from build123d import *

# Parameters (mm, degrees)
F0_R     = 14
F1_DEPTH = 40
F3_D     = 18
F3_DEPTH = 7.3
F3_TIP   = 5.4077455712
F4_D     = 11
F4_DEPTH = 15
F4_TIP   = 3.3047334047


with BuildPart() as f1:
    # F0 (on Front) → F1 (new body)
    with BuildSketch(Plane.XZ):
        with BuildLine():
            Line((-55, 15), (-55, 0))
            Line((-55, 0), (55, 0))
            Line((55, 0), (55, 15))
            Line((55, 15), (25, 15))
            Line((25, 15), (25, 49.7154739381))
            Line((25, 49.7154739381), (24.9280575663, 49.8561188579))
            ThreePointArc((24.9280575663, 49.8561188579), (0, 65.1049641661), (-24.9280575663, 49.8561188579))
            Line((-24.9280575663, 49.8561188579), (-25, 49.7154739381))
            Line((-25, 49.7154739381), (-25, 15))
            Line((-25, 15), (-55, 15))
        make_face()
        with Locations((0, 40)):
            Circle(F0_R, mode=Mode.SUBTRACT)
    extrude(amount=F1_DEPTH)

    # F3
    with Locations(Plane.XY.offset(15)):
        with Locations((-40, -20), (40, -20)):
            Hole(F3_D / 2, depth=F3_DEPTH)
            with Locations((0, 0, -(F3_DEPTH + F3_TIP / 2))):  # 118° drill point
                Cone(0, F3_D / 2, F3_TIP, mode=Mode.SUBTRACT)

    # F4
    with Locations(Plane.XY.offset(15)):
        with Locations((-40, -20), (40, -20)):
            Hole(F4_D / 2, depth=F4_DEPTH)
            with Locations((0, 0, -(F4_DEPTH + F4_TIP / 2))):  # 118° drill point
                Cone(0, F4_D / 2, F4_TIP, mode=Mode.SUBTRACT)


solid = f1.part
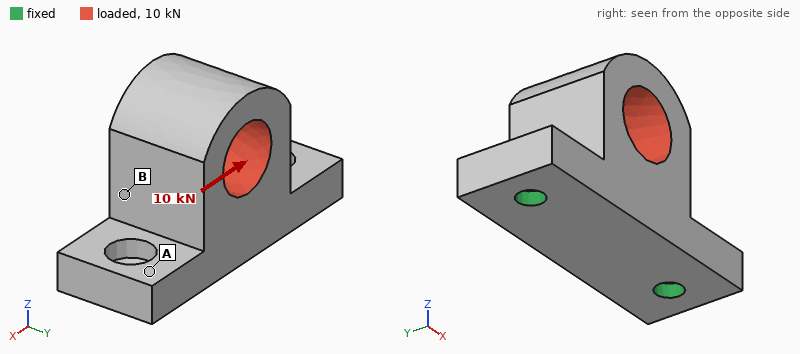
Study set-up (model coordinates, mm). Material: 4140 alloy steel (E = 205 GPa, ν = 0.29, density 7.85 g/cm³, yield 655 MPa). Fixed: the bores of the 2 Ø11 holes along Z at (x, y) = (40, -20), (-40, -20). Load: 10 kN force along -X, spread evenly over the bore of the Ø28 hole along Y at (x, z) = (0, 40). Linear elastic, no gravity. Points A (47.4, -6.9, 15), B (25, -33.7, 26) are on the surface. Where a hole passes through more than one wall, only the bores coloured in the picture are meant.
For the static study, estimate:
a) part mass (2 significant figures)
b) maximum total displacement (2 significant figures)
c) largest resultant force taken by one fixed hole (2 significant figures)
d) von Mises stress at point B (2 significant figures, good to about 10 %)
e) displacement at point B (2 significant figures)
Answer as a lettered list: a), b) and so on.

a) 1000 g
b) 19 µm
c) 7.1 kN
d) 23 MPa
e) 7.6 µm
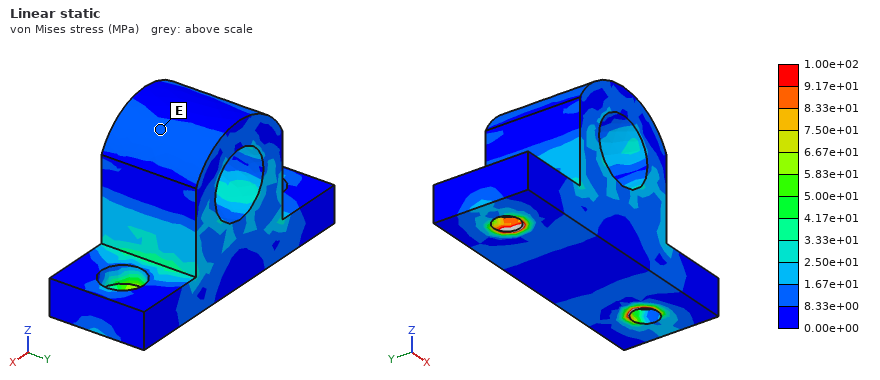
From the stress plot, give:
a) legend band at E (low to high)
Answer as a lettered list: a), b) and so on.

a) 8.33e+00 to 1.67e+01 MPa
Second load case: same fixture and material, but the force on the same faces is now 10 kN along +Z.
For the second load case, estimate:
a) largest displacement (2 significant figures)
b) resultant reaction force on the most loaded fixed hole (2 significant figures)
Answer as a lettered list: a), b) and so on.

a) 8.4 µm
b) 6.2 kN
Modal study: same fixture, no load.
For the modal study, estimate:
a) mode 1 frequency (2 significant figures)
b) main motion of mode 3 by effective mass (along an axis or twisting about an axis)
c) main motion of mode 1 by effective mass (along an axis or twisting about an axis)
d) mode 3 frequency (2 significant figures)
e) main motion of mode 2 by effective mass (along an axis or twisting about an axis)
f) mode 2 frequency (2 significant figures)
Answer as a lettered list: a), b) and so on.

a) 1900 Hz
b) along Z
c) along Y
d) 6700 Hz
e) along X
f) 5800 Hz
